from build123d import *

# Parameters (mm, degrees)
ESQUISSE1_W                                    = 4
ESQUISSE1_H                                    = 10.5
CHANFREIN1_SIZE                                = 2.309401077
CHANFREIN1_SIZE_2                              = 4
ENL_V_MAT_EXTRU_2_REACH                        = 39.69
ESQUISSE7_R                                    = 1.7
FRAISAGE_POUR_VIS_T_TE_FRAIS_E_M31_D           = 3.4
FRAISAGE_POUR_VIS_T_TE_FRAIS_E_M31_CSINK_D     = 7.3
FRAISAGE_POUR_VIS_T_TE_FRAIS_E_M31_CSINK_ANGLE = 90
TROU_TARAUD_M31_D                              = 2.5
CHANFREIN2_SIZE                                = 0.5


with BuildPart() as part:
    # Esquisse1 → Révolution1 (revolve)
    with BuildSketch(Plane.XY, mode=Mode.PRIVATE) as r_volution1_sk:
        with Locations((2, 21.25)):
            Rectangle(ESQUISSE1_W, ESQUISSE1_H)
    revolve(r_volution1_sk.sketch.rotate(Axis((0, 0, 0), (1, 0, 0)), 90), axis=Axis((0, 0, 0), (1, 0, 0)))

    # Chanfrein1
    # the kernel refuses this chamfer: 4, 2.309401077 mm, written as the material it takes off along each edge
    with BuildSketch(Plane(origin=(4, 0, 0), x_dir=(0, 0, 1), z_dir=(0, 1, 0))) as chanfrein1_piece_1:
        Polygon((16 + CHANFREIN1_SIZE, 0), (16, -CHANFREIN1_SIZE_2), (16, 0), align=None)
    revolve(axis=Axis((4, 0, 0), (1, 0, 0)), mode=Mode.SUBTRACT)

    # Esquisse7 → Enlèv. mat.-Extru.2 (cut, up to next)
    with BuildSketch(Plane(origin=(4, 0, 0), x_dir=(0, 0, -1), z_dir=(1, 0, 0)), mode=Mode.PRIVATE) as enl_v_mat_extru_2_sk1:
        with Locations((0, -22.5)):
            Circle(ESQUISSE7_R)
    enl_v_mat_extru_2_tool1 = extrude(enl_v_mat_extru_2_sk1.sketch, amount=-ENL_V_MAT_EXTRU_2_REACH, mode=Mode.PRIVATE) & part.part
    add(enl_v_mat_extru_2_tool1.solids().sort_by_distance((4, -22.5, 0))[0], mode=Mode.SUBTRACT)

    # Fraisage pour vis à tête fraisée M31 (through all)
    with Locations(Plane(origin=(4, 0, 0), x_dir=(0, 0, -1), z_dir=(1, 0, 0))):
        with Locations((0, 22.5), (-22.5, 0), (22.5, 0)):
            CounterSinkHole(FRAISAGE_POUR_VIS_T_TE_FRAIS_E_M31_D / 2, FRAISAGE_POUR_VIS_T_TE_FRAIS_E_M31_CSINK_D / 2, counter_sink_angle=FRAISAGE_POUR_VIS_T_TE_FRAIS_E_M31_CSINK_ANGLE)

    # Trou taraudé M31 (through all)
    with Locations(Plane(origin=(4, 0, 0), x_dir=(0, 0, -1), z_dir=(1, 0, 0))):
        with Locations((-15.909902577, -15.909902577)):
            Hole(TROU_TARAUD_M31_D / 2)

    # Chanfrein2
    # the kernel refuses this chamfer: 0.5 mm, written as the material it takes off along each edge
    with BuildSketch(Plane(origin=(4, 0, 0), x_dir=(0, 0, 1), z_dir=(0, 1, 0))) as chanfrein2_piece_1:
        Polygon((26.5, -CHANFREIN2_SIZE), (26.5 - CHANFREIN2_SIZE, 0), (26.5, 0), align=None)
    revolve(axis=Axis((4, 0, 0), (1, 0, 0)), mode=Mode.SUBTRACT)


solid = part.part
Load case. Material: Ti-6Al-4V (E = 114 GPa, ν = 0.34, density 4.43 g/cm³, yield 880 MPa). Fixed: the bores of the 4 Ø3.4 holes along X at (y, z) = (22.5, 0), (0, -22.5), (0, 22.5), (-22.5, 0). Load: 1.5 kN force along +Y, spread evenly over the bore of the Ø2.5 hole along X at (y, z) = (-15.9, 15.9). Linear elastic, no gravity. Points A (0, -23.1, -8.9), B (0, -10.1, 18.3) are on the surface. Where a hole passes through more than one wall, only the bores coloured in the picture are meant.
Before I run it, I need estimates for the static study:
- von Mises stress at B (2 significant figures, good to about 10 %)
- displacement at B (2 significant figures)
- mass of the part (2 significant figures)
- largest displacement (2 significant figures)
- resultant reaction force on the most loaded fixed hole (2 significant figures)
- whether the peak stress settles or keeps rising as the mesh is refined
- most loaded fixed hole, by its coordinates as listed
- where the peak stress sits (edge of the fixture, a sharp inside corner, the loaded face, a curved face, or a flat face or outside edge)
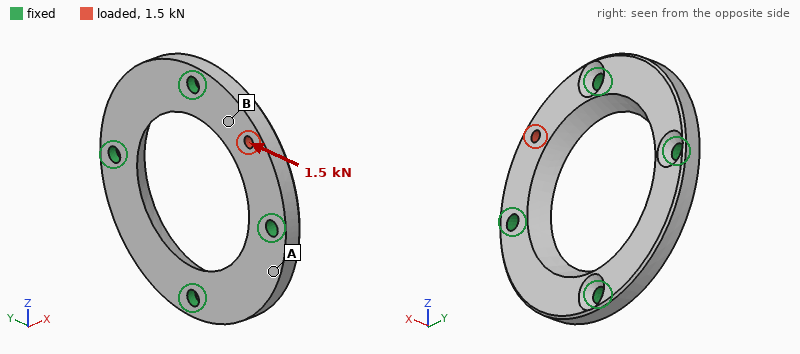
52 MPa
6.7 µm
21 g
12 µm
1.3 kN
keeps rising
(0, 22.5)
edge of the fixture
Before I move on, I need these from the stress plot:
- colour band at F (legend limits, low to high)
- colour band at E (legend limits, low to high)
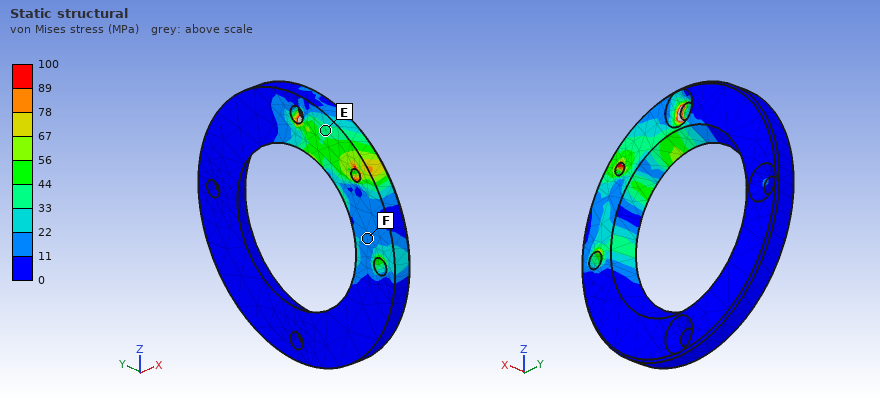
11 to 22 MPa
33 to 44 MPa
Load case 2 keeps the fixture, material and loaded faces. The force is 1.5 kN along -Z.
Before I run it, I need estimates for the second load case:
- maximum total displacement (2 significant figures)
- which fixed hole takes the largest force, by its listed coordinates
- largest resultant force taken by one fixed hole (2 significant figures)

11 µm
(-22.5, 0)
1.3 kN
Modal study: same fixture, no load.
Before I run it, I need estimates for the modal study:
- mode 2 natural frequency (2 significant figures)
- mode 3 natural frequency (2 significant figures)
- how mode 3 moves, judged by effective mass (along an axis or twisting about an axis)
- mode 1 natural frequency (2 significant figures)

13 kHz
14 kHz
twisting about Y
12 kHz
